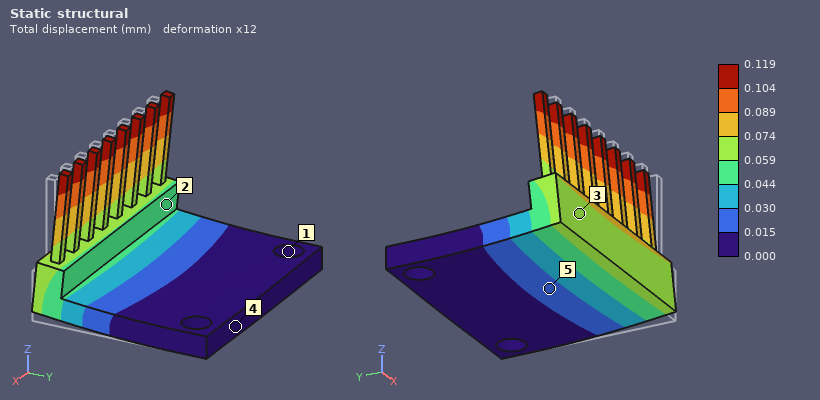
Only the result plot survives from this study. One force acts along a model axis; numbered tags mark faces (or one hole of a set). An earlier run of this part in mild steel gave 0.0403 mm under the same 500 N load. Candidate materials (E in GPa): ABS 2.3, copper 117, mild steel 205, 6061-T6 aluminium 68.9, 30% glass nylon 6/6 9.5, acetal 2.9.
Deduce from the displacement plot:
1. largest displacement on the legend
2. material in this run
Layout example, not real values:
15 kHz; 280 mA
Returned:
0.119 mm; 6061-T6 aluminium
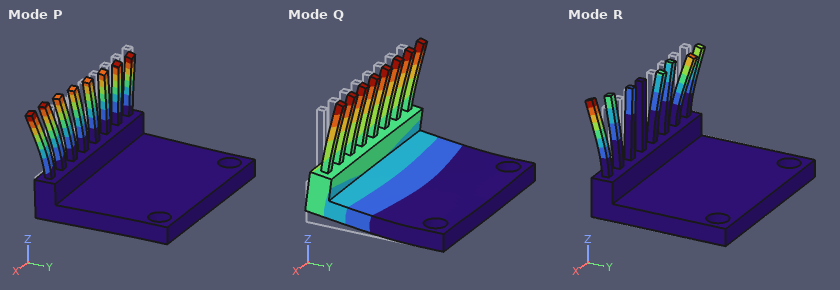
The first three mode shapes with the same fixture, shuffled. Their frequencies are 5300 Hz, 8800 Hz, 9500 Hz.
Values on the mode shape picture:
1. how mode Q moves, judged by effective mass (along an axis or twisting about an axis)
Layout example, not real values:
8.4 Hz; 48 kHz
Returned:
along Z
